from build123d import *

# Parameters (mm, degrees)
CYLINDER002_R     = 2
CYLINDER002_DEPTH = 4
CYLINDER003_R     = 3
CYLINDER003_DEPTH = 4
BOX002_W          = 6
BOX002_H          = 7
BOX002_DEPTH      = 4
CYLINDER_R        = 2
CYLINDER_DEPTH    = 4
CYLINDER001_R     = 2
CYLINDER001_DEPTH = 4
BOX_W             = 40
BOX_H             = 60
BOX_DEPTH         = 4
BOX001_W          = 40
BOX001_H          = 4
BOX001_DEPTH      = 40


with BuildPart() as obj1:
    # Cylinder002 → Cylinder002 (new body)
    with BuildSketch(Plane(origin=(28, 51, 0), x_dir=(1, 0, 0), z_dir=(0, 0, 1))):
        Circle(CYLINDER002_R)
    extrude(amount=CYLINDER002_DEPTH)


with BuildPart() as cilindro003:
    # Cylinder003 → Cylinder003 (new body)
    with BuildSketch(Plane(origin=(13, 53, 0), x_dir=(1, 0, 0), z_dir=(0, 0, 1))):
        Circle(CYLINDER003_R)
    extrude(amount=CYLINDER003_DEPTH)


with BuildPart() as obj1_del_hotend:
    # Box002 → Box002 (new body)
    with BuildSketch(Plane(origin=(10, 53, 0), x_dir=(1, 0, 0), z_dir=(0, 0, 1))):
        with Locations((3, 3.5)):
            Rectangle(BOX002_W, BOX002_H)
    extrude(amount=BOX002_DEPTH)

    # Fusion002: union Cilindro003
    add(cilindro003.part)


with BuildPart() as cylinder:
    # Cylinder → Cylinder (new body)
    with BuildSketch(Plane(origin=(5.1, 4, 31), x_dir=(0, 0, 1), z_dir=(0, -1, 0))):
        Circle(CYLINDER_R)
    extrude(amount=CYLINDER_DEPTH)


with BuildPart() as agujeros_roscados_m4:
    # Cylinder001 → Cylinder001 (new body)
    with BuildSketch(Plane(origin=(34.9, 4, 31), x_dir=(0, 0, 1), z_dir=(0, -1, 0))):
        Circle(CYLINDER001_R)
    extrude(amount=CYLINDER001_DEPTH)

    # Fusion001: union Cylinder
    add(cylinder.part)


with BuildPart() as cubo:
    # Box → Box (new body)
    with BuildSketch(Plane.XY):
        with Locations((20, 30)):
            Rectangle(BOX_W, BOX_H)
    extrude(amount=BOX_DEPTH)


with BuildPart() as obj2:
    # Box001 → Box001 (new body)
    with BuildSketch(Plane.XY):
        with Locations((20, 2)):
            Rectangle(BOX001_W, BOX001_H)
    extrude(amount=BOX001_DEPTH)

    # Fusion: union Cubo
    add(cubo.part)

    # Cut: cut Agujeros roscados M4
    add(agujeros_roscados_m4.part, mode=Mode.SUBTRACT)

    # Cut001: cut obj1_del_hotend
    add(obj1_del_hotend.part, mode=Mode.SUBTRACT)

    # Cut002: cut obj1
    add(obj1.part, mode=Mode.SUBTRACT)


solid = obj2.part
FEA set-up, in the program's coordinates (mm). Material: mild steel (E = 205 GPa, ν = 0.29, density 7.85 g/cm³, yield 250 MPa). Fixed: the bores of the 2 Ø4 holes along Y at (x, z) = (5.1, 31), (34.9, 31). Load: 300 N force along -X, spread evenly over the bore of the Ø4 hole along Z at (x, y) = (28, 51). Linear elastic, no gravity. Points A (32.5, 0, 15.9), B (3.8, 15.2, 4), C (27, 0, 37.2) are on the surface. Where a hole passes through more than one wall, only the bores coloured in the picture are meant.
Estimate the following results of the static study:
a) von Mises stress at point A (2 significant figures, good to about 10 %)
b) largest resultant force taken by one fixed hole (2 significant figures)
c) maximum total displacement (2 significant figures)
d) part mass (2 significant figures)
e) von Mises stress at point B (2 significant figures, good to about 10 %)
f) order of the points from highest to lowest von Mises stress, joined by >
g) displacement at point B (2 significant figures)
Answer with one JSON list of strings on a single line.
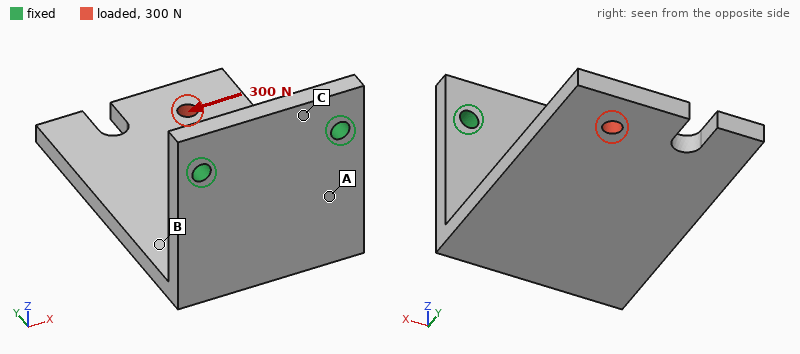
["79 MPa", "570 N", "0.22 mm", "120 g", "32 MPa", "A > B > C", "0.073 mm"]
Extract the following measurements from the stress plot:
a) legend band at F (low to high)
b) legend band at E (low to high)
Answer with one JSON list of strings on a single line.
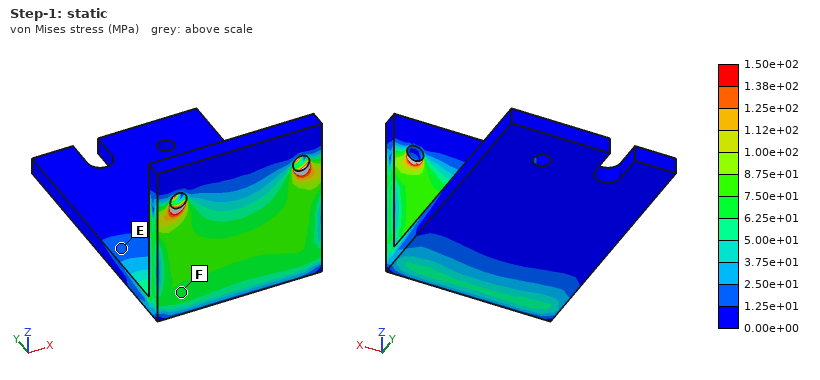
["6.25e+01 to 7.50e+01 MPa", "1.25e+01 to 2.50e+01 MPa"]
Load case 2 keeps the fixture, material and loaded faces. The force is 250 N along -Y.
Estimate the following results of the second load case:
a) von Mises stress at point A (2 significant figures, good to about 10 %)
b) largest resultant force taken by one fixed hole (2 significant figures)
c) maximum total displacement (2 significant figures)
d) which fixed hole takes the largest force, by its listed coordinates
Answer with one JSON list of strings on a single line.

["37 MPa", "190 N", "0.16 mm", "(34.9, 31)"]
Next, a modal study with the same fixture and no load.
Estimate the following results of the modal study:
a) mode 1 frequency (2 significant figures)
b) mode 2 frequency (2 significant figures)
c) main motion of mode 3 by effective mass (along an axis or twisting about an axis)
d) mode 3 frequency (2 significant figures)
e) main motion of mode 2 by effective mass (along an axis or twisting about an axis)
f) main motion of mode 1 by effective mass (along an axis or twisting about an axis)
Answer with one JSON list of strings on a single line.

["570 Hz", "1100 Hz", "along Y", "1900 Hz", "along X", "along Z"]
